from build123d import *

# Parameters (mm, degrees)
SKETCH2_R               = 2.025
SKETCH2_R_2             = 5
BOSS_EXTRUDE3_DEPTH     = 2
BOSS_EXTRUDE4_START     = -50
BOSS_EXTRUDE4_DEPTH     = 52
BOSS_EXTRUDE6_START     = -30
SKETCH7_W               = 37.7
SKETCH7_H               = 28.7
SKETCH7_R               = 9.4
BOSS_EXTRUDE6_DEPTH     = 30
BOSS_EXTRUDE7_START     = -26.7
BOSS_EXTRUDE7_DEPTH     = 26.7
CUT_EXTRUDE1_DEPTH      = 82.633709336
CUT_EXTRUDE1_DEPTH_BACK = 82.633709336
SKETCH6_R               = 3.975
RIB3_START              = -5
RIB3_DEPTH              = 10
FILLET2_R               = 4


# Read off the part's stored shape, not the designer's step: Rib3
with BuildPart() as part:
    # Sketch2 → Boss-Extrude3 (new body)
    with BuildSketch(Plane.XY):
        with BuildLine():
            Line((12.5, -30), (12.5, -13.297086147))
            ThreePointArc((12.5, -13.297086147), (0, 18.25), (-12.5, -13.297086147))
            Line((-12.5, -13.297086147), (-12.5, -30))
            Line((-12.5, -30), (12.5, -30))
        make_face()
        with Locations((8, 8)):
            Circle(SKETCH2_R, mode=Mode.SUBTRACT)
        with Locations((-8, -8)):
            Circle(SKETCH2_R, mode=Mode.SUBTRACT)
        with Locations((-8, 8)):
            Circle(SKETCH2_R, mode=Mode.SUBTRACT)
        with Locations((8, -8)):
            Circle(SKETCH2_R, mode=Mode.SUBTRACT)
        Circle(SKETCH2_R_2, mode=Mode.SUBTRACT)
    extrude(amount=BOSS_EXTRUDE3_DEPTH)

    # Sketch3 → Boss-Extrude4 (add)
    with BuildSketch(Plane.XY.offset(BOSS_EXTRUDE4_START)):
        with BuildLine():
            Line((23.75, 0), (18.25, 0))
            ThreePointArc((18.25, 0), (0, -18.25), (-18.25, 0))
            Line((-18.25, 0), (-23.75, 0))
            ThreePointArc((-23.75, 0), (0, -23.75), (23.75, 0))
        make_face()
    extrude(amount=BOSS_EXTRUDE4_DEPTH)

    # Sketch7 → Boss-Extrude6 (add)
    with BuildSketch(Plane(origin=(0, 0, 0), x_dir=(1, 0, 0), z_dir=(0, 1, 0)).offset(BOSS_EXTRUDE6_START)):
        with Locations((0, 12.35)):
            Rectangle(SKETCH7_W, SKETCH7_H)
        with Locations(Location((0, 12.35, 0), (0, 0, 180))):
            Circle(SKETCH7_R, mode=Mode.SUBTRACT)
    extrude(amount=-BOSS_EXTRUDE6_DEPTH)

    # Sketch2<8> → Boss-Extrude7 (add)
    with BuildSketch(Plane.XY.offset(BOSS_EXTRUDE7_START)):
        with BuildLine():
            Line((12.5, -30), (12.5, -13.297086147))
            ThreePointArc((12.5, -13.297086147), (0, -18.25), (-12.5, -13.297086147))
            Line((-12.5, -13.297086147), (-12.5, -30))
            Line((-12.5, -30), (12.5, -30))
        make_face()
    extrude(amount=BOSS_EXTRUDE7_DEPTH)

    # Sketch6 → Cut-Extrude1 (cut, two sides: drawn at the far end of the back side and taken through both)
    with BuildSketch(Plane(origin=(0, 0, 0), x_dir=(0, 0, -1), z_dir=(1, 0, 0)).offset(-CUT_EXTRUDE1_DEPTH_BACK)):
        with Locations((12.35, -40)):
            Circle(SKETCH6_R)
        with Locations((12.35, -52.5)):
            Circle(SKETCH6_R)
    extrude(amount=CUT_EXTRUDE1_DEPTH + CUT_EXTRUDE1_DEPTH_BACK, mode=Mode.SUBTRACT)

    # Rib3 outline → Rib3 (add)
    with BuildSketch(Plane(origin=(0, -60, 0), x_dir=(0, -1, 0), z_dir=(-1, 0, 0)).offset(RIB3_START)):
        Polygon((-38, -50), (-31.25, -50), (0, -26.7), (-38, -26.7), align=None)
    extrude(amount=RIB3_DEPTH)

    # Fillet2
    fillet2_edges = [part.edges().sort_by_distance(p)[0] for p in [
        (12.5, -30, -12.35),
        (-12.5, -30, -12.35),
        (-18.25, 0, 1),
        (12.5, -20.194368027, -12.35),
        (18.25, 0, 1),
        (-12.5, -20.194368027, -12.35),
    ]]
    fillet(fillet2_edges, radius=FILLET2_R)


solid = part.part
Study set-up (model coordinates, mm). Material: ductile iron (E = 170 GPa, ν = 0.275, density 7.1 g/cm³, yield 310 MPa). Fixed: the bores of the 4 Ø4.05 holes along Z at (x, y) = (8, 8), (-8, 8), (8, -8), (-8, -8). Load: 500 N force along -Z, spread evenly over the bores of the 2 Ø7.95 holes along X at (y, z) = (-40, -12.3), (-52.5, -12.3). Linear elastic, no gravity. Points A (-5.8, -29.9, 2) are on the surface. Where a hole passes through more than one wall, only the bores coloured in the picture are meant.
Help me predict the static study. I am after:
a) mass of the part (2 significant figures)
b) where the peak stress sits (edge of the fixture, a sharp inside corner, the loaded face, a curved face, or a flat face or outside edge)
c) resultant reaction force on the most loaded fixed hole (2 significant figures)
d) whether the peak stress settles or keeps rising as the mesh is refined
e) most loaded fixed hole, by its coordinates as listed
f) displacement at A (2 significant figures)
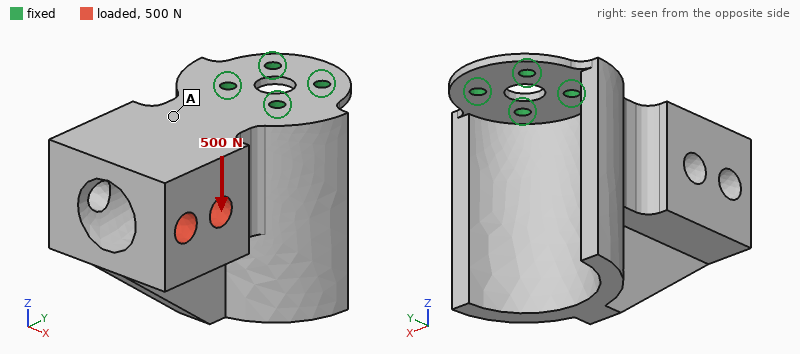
380 g
edge of the fixture
850 N
keeps rising
(8, -8)
0.13 mm
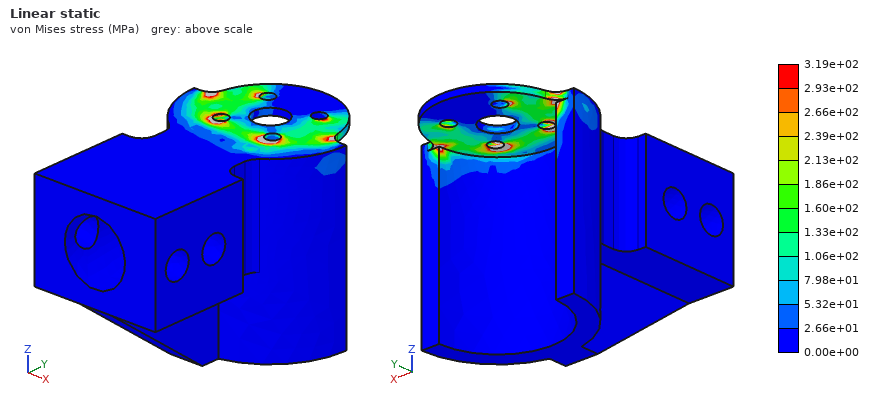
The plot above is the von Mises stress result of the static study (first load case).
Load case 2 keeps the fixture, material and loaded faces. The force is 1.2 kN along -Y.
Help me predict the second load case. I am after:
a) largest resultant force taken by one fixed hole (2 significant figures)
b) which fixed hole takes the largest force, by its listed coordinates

1.0 kN
(8, -8)
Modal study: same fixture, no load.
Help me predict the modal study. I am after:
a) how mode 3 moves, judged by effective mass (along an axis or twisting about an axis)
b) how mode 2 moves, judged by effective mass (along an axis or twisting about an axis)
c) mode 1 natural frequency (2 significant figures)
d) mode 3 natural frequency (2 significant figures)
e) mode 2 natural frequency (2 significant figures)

along X
along X
390 Hz
2700 Hz
1100 Hz
